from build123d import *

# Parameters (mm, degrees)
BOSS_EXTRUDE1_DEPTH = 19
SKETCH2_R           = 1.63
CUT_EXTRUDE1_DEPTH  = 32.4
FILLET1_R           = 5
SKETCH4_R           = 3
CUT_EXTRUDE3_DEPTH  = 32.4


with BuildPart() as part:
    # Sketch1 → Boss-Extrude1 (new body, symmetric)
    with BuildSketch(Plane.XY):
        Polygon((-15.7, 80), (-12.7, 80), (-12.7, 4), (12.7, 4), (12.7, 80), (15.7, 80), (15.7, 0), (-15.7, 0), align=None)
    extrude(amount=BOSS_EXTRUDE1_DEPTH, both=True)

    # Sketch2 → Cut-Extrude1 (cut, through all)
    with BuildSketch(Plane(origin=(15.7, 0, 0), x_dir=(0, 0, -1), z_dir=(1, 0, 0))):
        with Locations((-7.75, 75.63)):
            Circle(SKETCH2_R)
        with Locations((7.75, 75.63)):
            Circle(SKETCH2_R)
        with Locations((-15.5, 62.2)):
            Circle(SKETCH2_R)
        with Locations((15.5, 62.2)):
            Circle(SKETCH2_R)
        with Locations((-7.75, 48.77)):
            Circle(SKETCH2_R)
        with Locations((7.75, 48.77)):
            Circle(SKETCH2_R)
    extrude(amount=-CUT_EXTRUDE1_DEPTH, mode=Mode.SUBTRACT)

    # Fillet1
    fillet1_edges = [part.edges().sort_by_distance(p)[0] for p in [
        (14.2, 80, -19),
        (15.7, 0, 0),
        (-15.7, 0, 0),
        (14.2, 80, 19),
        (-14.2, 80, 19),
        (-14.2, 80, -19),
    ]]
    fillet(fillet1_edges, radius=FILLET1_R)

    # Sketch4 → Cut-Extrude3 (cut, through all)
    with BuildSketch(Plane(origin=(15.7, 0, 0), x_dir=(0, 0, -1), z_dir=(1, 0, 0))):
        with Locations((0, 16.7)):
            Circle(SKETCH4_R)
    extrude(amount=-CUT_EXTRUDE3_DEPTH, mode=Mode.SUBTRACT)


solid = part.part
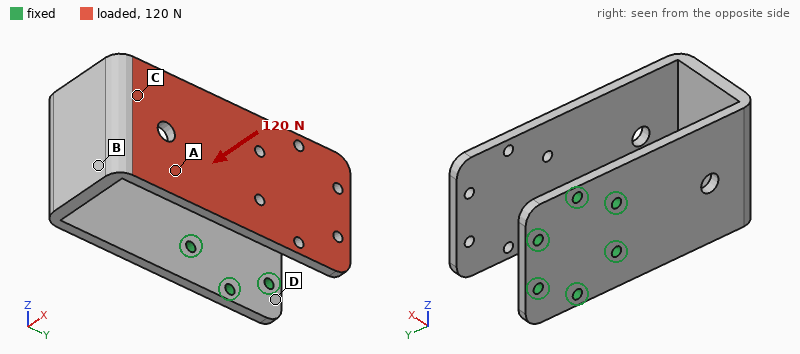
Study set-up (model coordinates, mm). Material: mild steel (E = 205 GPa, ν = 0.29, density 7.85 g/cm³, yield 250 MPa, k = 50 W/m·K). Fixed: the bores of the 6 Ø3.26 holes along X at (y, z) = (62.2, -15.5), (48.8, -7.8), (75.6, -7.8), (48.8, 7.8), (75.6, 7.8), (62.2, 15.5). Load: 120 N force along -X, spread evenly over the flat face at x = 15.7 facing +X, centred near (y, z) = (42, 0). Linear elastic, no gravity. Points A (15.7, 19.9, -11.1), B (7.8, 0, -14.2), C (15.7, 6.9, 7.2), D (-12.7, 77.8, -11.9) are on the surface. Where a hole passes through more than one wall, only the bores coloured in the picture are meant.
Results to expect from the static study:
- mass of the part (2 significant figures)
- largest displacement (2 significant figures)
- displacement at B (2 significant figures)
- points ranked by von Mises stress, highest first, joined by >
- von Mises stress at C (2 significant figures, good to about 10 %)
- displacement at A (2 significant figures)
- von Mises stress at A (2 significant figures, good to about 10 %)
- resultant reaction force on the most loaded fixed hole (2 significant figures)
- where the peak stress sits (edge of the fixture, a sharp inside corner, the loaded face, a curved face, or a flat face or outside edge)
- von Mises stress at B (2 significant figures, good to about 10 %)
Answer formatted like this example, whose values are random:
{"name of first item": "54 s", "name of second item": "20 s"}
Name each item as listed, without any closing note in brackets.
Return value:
{"mass of the part": "170 g", "largest displacement": "1.0 mm", "displacement at B": "0.17 mm", "points ranked by von Mises stress, highest first, joined by >": "C > A > B > D", "von Mises stress at C": "65 MPa", "displacement at A": "0.25 mm", "von Mises stress at A": "53 MPa", "resultant reaction force on the most loaded fixed hole": "65 N", "where the peak stress sits": "a curved face", "von Mises stress at B": "42 MPa"}
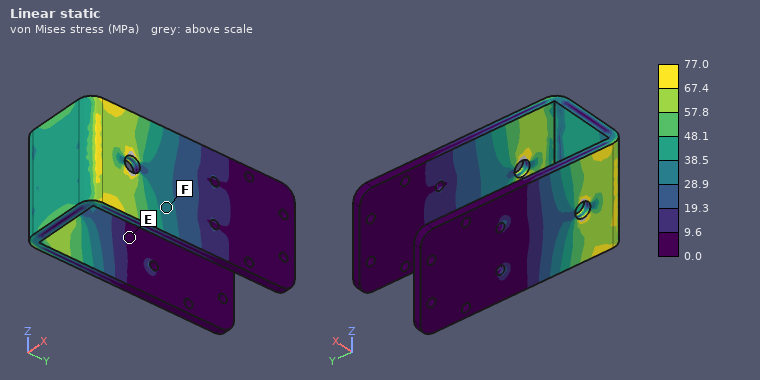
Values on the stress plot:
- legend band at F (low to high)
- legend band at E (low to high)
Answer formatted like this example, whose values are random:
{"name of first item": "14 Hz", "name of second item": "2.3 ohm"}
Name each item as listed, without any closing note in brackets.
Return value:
{"legend band at F": "28.9 to 38.5 MPa", "legend band at E": "0.0 to 9.6 MPa"}
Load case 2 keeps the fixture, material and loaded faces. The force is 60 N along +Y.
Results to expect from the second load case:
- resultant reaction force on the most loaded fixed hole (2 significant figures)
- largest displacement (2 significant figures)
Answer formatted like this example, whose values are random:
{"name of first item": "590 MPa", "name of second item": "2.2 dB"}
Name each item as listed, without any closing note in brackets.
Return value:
{"resultant reaction force on the most loaded fixed hole": "33 N", "largest displacement": "0.35 mm"}
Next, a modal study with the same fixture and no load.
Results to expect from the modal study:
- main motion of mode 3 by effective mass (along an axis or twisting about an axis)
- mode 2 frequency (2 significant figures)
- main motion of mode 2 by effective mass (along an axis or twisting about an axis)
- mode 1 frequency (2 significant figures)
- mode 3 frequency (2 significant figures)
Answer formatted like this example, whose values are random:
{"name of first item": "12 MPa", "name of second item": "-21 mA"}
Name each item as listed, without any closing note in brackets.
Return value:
{"main motion of mode 3 by effective mass": "along X", "mode 2 frequency": "400 Hz", "main motion of mode 2 by effective mass": "along Z", "mode 1 frequency": "230 Hz", "mode 3 frequency": "430 Hz"}
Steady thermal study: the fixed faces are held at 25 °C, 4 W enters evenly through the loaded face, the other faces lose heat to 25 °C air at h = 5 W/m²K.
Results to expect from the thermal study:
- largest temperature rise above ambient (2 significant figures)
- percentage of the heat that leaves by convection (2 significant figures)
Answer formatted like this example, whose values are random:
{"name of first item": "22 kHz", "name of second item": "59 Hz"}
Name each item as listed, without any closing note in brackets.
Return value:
{"largest temperature rise above ambient": "55 K", "percentage of the heat that leaves by convection": "36 %"}
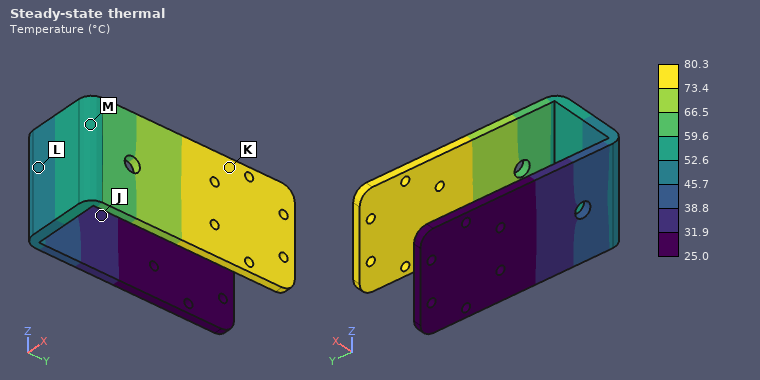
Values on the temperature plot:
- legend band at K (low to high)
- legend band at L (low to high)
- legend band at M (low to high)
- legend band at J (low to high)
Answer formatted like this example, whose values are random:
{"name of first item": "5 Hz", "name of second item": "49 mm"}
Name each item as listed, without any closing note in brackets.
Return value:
{"legend band at K": "73.4 to 80.3 °C", "legend band at L": "45.7 to 52.6 °C", "legend band at M": "52.6 to 59.6 °C", "legend band at J": "31.9 to 38.8 °C"}
